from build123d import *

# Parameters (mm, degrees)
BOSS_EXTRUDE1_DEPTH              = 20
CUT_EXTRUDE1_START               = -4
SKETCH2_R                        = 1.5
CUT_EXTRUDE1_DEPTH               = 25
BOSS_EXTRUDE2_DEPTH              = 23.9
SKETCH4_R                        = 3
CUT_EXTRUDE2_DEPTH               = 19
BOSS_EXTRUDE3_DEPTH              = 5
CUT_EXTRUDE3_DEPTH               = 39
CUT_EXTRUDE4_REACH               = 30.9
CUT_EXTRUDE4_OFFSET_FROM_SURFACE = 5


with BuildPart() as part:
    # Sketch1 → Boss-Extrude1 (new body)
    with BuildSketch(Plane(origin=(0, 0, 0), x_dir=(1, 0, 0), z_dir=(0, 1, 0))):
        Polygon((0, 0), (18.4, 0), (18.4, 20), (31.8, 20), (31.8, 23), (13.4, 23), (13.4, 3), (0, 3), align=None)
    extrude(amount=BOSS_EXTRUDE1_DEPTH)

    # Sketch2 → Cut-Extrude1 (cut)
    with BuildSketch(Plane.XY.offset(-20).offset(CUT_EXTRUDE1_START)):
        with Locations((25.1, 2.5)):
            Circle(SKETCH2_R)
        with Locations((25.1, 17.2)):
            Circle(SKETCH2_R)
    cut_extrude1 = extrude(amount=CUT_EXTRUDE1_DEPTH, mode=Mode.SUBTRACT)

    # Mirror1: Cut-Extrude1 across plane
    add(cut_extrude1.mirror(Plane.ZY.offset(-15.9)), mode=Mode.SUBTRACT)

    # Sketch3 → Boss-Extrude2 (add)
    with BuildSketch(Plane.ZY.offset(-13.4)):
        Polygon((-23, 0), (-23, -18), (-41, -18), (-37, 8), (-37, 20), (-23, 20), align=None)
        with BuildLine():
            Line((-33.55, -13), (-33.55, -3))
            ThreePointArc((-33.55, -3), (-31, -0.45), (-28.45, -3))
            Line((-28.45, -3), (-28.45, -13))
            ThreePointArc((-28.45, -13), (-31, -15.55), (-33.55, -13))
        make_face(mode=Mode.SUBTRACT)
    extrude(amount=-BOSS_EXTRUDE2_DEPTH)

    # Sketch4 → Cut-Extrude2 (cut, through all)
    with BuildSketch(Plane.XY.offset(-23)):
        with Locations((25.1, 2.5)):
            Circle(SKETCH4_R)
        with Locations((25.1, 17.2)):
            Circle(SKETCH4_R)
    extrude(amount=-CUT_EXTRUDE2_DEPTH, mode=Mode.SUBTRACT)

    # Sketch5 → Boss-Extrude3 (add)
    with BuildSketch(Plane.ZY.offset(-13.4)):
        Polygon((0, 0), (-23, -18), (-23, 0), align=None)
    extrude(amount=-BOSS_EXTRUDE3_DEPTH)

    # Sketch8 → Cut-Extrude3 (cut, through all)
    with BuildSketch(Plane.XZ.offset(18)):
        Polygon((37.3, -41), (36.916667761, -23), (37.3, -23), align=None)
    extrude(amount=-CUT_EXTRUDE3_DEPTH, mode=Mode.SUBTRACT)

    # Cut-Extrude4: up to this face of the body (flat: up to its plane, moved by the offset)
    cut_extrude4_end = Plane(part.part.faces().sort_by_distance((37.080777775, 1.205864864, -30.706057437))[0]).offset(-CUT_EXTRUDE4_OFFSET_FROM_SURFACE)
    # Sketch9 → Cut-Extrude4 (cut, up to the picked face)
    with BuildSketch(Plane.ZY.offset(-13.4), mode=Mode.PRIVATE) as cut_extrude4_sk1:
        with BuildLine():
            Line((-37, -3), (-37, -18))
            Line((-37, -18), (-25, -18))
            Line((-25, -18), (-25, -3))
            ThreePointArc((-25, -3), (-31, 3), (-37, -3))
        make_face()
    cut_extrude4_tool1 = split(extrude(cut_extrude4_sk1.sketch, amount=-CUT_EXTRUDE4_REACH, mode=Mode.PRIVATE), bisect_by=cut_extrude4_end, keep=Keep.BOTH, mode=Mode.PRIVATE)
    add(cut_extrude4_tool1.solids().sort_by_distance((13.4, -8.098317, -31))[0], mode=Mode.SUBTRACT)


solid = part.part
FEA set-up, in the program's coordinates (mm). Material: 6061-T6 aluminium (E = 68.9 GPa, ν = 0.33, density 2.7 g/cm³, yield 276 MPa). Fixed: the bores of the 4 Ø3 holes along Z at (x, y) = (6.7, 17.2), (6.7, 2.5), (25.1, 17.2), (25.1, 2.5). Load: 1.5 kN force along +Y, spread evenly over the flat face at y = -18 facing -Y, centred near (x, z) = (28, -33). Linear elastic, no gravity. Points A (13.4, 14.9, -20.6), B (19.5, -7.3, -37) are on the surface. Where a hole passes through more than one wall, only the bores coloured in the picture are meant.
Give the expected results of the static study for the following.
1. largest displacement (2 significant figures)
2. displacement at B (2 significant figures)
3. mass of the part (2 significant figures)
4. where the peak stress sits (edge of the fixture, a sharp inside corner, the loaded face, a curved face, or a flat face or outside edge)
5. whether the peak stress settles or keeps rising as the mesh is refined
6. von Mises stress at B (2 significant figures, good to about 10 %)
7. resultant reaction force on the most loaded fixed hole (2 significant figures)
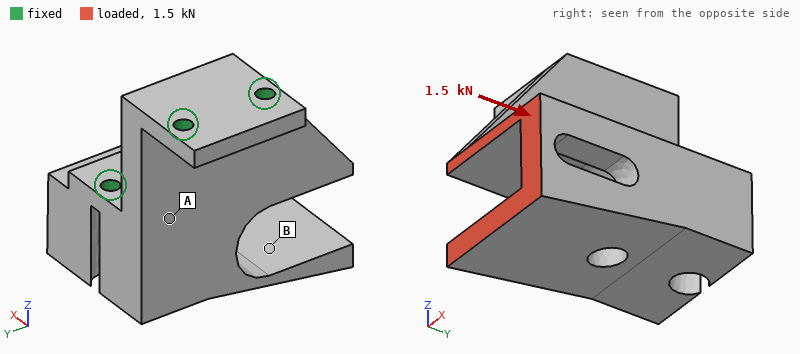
65 µm
31 µm
36 g
edge of the fixture
keeps rising
19 MPa
1.2 kN
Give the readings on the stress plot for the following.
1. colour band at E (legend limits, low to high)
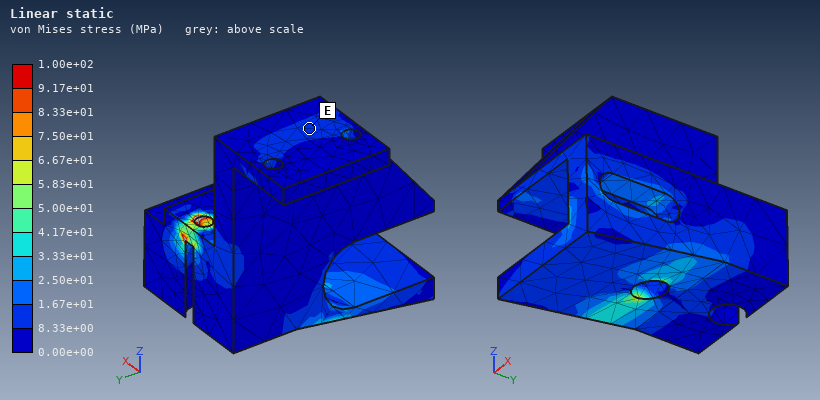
8.33e+00 to 1.67e+01 MPa
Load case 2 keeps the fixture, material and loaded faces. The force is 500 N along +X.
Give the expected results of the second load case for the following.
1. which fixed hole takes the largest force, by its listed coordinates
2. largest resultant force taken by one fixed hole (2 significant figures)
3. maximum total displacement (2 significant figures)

(25.1, 2.5)
1.1 kN
46 µm
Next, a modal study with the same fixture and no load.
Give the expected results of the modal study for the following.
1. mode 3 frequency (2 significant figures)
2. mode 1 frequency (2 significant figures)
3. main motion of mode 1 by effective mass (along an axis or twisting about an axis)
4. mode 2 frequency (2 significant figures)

11 kHz
6000 Hz
along X
6300 Hz
